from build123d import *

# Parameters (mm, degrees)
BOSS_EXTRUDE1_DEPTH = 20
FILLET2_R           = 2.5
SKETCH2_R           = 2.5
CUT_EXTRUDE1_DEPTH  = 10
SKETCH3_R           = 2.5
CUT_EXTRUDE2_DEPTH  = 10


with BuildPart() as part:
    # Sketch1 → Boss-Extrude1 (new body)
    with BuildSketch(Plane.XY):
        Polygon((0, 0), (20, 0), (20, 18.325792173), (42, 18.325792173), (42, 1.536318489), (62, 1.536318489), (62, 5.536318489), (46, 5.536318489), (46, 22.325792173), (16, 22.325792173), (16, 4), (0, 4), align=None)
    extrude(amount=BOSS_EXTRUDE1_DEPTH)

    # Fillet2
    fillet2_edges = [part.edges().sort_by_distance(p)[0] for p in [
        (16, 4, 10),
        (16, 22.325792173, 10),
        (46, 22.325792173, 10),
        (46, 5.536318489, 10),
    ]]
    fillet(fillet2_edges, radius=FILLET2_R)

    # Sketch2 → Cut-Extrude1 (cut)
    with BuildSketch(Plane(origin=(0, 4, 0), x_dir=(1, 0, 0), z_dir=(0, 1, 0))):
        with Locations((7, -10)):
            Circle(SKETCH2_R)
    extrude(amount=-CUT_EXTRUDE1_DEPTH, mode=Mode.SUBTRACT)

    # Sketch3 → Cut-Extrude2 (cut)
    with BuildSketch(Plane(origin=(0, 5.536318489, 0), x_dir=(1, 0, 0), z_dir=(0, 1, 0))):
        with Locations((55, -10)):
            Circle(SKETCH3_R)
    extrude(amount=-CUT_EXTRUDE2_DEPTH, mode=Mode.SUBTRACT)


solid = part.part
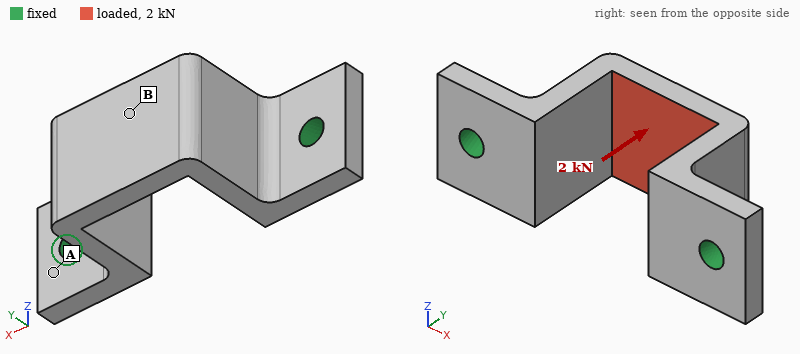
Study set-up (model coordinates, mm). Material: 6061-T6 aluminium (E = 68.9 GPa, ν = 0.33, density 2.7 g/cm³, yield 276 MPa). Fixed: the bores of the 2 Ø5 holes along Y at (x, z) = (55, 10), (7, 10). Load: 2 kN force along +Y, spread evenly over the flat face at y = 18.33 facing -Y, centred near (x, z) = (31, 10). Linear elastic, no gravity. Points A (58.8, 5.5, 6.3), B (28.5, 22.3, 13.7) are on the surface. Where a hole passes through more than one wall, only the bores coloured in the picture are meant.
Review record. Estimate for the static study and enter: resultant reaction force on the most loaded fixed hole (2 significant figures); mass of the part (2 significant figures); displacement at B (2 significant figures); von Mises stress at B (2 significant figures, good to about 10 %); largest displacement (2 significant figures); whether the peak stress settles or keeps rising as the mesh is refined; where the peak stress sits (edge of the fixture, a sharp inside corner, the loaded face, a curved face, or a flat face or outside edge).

1.2 kN
21 g
42 µm
53 MPa
47 µm
keeps rising
edge of the fixture
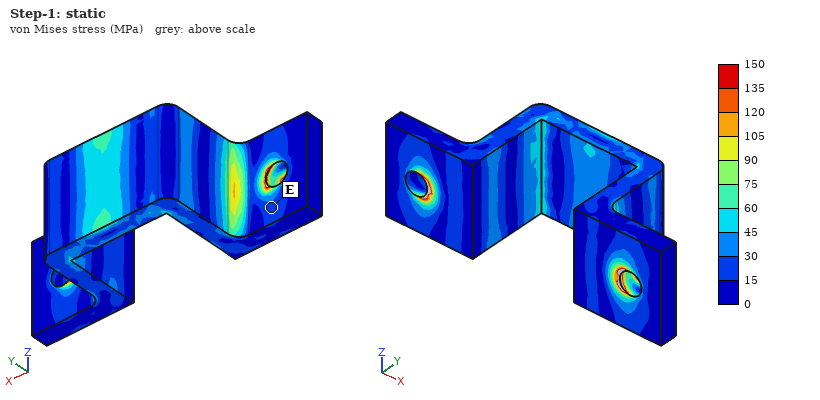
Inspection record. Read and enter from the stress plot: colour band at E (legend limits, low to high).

15 to 30 MPa
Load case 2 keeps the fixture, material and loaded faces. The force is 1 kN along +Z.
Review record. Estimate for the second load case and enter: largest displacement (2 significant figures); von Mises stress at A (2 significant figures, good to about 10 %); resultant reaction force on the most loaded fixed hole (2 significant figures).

0.13 mm
34 MPa
520 N
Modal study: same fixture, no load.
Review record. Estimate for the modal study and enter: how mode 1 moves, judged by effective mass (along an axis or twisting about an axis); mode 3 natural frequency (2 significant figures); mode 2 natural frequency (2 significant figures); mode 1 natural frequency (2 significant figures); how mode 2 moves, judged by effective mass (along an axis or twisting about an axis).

along Z
9300 Hz
7100 Hz
4800 Hz
along X
